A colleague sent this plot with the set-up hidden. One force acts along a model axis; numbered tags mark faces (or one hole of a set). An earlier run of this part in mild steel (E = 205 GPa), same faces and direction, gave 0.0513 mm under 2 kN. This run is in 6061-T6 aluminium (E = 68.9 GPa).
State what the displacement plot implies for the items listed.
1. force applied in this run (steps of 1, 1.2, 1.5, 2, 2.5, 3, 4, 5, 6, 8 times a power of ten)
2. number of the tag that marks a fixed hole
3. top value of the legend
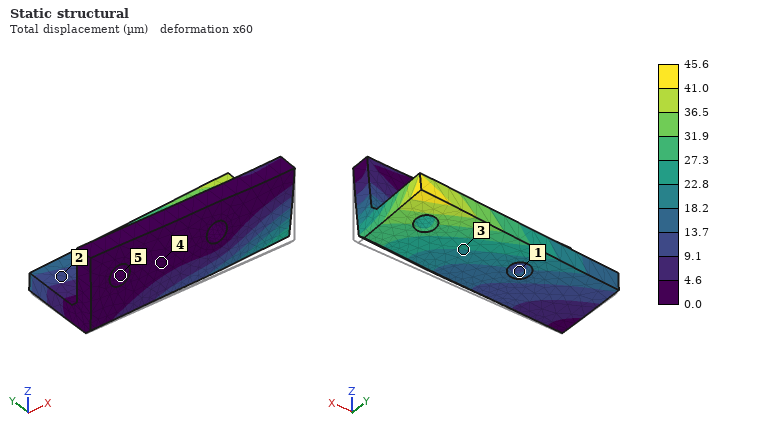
600 N
5
45.6 µm
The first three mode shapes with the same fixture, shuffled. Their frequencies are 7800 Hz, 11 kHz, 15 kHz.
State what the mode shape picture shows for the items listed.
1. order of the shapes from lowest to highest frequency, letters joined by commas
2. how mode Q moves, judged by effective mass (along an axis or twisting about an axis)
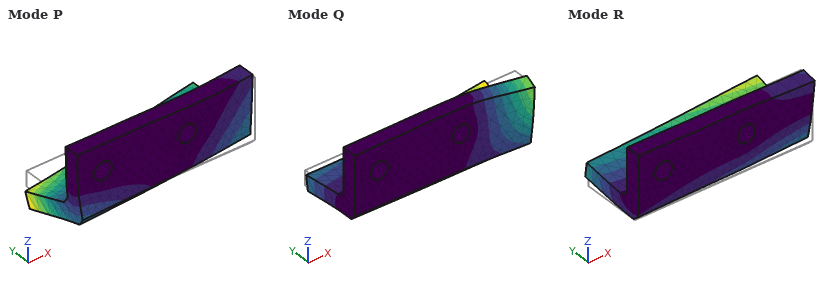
R, P, Q
along Y
